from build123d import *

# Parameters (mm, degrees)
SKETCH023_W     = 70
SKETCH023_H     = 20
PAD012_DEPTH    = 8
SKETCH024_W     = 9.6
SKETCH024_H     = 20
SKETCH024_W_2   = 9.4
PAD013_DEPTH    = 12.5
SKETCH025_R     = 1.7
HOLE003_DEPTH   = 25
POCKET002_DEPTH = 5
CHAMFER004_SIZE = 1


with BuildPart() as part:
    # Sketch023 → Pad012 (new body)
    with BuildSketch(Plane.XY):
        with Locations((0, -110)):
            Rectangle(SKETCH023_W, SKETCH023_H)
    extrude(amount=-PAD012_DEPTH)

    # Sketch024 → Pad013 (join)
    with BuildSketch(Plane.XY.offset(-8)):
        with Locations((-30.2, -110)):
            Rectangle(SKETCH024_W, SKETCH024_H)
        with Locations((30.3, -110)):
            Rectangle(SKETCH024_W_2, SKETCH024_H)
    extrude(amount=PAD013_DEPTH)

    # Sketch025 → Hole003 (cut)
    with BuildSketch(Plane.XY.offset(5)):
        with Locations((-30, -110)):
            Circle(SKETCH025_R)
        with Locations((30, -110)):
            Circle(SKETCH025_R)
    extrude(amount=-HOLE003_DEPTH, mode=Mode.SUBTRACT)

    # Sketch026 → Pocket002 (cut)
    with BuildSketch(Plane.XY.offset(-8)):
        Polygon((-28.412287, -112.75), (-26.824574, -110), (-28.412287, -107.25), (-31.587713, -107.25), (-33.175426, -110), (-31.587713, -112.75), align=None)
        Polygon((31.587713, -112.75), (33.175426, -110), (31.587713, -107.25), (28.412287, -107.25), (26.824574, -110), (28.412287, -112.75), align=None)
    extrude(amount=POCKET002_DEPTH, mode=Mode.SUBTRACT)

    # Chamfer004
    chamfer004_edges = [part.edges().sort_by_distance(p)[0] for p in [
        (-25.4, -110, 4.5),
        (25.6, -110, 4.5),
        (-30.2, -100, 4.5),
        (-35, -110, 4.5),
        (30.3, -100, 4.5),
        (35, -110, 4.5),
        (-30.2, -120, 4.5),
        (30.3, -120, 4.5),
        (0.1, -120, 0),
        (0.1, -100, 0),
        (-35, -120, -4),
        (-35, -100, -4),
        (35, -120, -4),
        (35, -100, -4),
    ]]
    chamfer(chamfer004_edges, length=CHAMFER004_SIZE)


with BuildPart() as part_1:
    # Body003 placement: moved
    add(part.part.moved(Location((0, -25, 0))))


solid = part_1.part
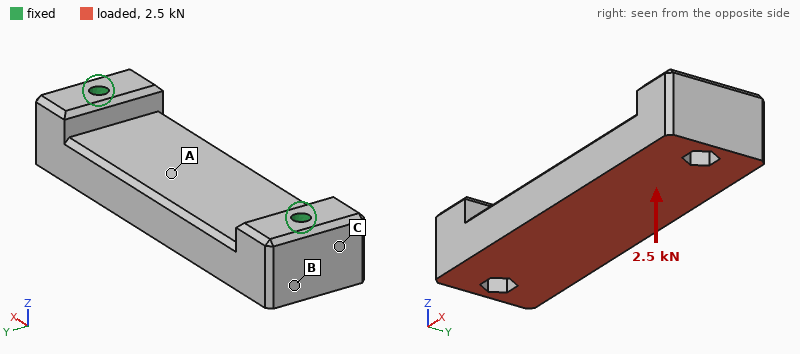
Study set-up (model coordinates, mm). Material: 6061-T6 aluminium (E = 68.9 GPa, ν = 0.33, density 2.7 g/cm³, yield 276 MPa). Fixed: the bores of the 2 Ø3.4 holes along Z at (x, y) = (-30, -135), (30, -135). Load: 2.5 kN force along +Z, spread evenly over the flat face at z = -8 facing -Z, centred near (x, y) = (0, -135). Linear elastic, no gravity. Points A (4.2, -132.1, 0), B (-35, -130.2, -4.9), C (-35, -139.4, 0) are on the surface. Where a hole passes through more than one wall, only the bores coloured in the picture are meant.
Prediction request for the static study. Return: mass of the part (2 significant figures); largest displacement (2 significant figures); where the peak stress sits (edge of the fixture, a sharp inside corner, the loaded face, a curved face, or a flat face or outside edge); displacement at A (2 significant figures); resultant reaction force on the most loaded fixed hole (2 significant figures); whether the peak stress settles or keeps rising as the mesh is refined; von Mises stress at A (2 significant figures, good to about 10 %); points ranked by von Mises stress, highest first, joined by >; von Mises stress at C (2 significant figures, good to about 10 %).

33 g
33 µm
edge of the fixture
31 µm
1.6 kN
keeps rising
22 MPa
A > C > B
14 MPa
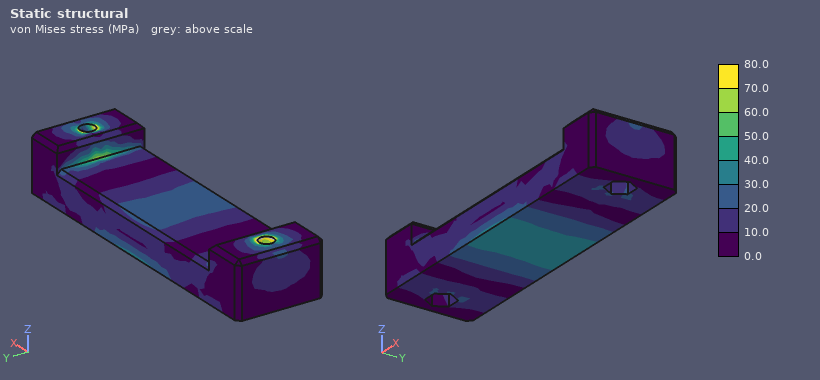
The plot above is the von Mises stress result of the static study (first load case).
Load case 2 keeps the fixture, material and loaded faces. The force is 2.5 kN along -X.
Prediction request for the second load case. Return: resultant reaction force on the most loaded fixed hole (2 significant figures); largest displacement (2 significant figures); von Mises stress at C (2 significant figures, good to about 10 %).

1.3 kN
5.3 µm
8.1 MPa
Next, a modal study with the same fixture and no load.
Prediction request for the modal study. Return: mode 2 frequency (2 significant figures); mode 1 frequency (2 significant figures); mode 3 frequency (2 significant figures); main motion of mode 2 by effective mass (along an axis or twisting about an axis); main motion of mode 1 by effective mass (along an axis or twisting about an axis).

11 kHz
9200 Hz
16 kHz
along Y
along Z
